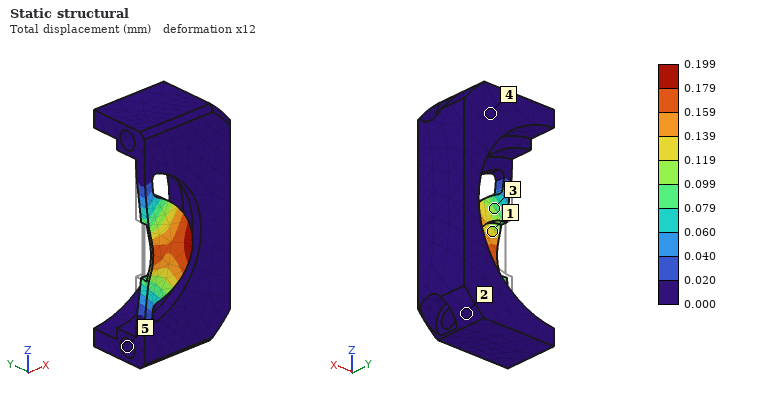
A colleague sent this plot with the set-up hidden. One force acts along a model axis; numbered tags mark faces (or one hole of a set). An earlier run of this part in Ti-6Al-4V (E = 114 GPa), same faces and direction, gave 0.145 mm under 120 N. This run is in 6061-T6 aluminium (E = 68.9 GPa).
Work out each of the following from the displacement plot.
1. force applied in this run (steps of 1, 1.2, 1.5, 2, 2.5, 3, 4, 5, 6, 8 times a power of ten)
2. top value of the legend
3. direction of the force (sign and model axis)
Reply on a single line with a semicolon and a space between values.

100 N; 0.199 mm; -Y
